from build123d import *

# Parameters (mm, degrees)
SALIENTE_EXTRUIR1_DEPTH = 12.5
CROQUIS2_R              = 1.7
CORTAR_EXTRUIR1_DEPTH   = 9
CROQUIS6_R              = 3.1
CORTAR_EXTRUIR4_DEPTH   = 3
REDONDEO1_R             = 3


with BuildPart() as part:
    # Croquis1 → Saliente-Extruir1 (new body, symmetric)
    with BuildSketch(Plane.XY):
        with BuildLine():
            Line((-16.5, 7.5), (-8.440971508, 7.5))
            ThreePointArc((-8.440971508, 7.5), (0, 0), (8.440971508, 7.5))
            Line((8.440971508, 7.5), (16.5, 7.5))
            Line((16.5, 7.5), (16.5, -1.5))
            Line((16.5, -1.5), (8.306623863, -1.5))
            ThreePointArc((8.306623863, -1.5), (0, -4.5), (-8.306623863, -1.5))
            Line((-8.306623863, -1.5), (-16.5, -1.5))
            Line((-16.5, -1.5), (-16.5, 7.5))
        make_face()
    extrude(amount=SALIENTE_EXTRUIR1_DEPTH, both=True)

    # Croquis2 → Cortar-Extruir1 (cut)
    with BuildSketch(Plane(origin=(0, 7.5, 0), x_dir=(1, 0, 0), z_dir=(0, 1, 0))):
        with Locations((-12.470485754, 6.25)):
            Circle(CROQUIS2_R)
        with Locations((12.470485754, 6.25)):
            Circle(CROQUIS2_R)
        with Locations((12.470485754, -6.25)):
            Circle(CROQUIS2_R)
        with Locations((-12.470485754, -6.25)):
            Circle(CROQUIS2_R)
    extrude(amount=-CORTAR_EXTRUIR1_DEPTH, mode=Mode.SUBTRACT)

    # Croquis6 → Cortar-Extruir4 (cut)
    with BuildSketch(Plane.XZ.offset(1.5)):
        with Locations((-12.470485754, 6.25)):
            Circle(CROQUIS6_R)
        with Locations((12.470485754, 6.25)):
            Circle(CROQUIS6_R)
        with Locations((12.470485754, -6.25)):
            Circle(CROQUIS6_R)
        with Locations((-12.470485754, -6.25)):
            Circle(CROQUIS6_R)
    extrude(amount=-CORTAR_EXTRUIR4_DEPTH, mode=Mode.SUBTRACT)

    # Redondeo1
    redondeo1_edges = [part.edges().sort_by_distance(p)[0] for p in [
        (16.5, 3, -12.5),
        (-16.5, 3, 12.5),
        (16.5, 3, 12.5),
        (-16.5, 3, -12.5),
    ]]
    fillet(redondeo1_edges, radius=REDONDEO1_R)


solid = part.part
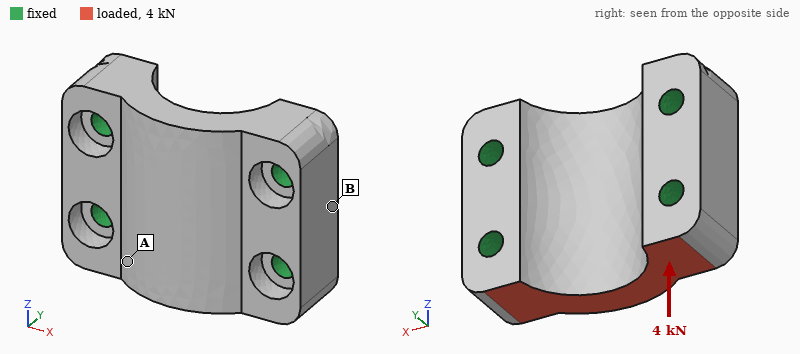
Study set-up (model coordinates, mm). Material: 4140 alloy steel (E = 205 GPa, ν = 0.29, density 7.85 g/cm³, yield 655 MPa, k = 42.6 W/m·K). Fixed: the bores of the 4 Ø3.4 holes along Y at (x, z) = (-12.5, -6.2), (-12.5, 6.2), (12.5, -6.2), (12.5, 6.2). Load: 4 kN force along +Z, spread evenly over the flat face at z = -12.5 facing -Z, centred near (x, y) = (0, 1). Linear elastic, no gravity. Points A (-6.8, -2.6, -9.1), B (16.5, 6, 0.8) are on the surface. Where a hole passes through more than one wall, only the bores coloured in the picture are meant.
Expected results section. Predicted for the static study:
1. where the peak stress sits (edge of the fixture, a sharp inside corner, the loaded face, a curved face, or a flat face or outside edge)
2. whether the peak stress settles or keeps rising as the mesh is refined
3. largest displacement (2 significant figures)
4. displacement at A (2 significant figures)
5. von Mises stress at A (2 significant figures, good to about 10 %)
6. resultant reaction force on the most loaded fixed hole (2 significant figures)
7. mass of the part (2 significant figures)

edge of the fixture
keeps rising
3.9 µm
2.5 µm
27 MPa
1.5 kN
41 g
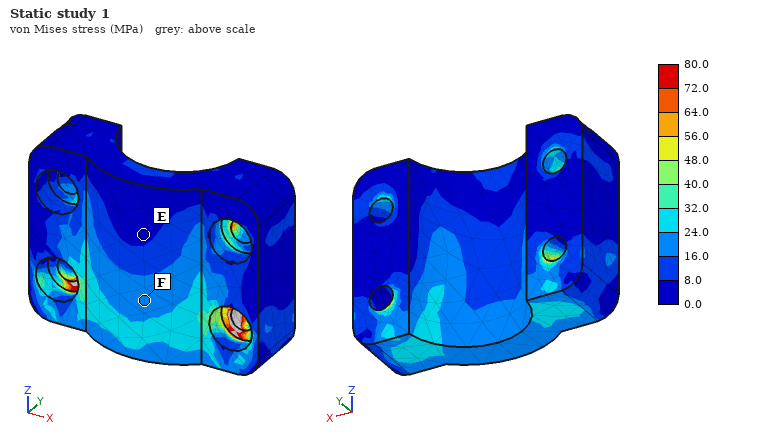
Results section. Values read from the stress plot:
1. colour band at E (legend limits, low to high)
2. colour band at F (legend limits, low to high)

0.0 to 8.0 MPa
16.0 to 24.0 MPa
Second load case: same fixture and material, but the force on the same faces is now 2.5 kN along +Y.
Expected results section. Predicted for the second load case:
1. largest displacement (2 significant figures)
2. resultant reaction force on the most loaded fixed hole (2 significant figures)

7.0 µm
1.6 kN
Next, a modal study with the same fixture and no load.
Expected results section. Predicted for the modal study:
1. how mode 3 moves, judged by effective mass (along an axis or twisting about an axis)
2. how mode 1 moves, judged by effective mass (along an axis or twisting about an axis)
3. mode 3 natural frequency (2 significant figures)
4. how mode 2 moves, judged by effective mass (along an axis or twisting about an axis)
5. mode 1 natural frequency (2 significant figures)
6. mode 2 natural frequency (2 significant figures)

along X
along Z
55 kHz
along Y
41 kHz
50 kHz
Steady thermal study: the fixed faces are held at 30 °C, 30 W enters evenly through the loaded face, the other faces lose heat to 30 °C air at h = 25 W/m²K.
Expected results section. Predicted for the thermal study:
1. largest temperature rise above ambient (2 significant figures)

42 K
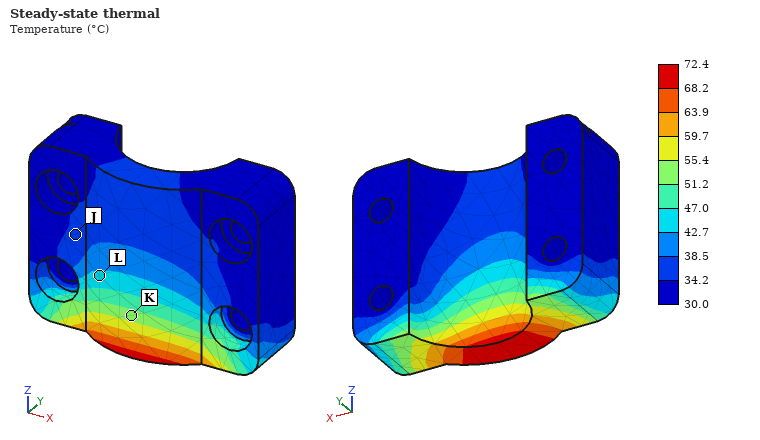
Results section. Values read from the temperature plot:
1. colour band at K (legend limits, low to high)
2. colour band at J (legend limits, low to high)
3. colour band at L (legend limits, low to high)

51.2 to 55.4 °C
34.2 to 38.5 °C
42.7 to 47.0 °C
